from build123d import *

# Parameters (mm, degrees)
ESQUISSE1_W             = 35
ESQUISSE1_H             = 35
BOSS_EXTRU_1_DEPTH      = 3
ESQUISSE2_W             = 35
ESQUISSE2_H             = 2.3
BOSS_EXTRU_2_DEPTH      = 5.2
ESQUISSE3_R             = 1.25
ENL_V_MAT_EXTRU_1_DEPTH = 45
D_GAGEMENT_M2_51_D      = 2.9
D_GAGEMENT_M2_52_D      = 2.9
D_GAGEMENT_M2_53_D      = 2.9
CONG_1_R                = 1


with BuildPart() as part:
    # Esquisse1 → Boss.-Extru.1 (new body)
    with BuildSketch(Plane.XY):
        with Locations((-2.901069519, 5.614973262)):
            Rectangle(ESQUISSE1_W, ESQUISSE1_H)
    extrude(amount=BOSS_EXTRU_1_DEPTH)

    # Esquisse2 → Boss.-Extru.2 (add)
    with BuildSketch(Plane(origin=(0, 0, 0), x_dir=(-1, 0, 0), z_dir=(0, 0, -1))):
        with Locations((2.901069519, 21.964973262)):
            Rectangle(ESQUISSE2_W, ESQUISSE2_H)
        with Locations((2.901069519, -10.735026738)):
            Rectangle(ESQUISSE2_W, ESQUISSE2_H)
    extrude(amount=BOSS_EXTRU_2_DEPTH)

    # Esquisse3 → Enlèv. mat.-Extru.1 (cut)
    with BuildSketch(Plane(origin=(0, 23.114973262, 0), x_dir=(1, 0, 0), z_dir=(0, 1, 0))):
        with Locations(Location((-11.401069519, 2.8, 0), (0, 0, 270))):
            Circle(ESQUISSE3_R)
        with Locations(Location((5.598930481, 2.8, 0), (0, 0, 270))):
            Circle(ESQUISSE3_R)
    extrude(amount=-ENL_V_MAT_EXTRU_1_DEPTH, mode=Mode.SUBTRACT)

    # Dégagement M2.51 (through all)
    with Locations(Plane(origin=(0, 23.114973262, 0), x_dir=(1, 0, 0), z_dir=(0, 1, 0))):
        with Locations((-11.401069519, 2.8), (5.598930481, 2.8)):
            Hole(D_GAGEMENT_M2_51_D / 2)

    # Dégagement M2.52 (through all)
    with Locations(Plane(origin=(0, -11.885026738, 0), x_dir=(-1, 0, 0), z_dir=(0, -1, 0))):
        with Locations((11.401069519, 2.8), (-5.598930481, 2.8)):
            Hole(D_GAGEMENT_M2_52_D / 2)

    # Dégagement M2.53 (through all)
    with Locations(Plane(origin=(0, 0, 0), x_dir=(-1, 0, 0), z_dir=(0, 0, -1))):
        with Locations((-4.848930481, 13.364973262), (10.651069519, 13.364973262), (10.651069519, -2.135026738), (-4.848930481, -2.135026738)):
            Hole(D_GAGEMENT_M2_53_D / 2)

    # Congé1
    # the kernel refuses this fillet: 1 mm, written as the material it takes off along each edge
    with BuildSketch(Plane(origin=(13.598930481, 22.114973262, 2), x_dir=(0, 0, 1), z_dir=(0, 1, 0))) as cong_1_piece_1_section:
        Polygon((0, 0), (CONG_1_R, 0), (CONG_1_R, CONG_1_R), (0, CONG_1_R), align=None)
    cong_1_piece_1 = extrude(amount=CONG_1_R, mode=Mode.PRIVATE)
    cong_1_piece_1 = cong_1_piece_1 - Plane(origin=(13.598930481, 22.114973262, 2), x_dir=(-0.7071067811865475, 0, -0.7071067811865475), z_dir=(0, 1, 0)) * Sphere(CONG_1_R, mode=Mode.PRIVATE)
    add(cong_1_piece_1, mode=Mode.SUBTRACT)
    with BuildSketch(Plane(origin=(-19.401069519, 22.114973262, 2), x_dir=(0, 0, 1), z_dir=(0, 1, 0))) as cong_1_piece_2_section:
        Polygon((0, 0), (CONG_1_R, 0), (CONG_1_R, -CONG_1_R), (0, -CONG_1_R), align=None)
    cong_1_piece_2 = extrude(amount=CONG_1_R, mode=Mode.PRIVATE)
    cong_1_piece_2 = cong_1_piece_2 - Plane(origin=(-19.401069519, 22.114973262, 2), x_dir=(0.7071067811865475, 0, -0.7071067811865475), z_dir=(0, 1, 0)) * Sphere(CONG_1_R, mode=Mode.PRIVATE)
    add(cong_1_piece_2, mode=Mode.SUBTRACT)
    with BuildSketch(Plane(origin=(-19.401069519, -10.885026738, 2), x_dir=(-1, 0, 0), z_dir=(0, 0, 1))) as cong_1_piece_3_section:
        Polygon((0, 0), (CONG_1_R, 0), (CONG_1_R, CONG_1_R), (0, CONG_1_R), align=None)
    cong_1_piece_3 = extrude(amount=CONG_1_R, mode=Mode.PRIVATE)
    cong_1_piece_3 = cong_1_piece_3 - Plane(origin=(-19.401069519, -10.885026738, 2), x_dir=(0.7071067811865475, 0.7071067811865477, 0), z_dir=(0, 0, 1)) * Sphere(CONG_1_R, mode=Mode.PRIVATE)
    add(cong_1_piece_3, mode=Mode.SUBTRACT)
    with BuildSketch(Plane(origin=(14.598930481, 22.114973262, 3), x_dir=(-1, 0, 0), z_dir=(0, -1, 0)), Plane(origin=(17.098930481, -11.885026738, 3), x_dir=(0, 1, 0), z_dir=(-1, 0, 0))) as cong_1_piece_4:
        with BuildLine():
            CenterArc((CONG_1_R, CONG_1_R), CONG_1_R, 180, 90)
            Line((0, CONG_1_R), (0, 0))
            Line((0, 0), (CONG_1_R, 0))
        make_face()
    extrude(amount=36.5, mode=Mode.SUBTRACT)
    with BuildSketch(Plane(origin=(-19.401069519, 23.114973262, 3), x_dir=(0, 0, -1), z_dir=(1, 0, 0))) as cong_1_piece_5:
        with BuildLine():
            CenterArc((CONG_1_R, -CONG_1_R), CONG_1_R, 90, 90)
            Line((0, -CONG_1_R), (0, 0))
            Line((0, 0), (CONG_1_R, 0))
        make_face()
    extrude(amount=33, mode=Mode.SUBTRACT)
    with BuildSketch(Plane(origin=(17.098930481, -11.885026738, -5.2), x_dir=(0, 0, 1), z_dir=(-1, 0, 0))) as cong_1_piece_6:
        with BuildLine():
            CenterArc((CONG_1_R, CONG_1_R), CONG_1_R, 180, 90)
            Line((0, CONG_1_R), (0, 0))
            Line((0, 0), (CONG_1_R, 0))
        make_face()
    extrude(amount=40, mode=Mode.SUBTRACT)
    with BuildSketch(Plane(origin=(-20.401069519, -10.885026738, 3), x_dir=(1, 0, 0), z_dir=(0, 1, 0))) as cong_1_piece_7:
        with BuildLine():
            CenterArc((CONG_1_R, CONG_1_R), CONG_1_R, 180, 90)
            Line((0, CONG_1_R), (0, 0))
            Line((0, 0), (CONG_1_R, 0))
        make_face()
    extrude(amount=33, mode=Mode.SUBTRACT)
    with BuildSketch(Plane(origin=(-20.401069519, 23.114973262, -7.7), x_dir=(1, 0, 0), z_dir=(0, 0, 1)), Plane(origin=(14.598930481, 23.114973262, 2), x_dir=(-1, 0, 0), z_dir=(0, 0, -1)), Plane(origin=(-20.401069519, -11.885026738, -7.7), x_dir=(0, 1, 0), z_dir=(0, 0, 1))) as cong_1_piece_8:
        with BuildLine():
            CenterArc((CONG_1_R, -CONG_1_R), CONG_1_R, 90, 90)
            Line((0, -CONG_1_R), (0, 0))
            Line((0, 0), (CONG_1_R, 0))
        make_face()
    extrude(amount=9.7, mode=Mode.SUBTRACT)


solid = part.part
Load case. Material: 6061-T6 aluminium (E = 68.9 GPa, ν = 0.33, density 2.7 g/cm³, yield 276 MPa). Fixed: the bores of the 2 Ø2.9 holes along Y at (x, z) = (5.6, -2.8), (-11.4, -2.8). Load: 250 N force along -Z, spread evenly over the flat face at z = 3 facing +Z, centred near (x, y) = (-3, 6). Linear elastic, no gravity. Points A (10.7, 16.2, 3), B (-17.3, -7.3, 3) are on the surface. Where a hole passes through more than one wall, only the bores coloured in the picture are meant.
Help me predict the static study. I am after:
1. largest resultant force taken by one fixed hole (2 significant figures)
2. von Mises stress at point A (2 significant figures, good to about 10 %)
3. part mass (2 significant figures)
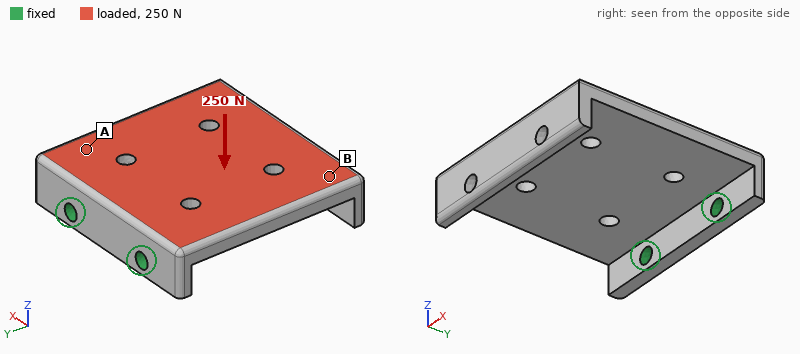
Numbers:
130 N
52 MPa
12 g
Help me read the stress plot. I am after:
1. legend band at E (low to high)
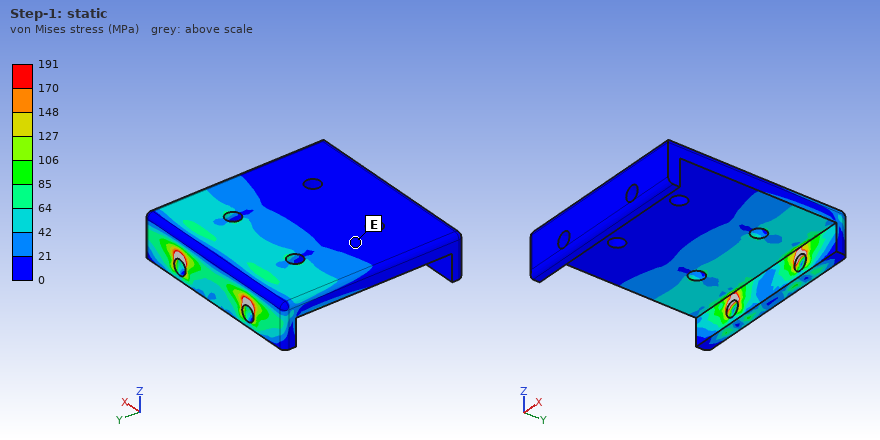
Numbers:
0 to 21 MPa
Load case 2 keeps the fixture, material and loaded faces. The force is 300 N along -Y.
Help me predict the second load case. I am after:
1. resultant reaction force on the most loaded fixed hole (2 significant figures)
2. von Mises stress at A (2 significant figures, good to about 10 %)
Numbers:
150 N
9.2 MPa
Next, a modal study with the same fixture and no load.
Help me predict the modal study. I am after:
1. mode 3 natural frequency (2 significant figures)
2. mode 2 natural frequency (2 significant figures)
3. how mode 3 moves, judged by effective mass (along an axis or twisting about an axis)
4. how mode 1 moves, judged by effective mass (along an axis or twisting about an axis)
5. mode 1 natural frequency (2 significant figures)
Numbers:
6000 Hz
3600 Hz
along X
along Z
1300 Hz
